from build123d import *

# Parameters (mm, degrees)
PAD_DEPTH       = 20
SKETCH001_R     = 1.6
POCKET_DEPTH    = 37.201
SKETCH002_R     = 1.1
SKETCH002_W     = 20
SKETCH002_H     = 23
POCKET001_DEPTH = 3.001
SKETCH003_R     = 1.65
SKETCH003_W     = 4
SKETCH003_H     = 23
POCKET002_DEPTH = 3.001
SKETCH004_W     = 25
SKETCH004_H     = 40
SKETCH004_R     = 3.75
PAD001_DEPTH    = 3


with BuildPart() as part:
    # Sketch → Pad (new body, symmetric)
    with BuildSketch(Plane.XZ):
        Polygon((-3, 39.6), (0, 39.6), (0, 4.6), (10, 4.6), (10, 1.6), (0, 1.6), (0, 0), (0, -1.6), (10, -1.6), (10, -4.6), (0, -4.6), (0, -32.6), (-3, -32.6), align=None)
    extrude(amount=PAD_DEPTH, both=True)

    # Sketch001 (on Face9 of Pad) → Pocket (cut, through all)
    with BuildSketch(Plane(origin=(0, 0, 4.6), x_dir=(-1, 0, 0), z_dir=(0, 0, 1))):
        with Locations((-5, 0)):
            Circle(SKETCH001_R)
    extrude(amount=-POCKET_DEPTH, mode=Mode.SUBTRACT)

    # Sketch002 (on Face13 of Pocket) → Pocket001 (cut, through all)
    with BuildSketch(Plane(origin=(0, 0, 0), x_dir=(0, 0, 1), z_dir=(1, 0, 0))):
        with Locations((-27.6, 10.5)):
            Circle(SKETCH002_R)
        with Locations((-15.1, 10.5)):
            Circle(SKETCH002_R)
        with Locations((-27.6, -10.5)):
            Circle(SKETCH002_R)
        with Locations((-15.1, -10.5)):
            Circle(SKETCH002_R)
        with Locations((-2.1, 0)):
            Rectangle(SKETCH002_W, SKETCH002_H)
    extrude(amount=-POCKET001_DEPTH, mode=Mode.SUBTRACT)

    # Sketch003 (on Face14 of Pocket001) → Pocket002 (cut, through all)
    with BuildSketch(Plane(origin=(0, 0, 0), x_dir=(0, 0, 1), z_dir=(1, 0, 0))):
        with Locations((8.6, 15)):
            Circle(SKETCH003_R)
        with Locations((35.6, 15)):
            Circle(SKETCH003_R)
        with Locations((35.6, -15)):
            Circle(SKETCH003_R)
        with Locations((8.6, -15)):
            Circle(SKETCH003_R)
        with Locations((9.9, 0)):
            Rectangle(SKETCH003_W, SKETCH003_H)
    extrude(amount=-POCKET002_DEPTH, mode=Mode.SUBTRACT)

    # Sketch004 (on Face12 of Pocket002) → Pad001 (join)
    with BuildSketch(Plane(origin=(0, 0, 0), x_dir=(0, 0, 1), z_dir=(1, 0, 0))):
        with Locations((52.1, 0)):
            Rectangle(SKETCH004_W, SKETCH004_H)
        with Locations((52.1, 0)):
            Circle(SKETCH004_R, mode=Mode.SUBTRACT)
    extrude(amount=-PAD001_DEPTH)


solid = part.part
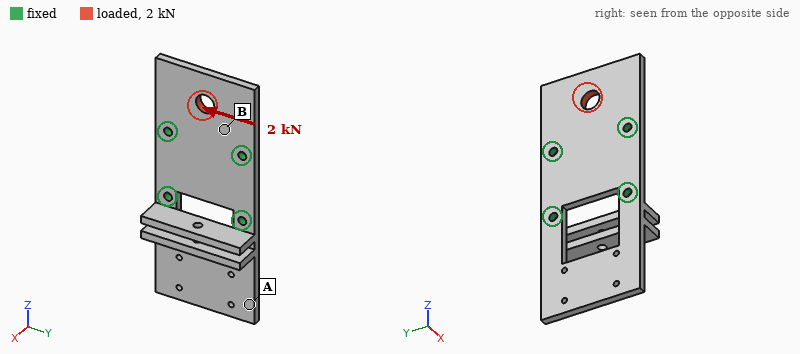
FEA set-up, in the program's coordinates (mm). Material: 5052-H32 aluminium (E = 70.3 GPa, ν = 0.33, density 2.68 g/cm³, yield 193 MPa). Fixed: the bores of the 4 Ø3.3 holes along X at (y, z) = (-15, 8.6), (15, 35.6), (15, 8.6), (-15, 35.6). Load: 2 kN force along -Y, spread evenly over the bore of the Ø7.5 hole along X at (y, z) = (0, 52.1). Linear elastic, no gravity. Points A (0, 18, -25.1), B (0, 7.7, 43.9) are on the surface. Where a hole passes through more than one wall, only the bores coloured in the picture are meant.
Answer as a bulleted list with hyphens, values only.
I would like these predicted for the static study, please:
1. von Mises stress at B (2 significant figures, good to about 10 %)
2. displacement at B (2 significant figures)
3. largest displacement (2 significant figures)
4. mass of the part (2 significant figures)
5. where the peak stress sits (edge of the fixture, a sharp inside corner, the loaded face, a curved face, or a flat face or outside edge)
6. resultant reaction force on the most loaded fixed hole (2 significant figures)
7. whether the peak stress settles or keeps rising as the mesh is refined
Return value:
- 35 MPa
- 8.0 µm
- 24 µm
- 32 g
- edge of the fixture
- 1.4 kN
- keeps rising
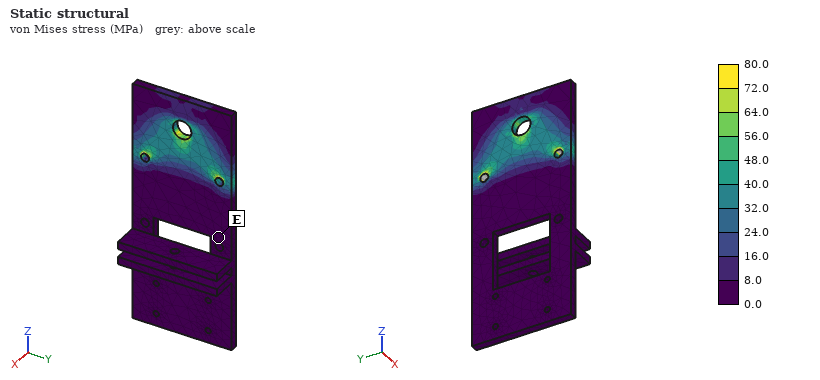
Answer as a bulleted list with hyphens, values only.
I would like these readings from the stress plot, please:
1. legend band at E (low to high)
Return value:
- 0.0 to 8.0 MPa
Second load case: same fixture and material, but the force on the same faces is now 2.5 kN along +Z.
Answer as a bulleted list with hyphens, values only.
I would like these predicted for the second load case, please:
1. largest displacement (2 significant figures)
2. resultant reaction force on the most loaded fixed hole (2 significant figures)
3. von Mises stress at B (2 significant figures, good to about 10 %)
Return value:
- 14 µm
- 1.1 kN
- 30 MPa
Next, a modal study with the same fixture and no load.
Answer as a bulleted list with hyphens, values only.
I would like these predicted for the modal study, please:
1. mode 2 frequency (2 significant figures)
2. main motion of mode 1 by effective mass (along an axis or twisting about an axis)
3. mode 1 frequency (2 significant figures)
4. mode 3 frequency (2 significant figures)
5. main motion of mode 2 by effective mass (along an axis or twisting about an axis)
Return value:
- 2800 Hz
- along X
- 1100 Hz
- 3400 Hz
- along X
